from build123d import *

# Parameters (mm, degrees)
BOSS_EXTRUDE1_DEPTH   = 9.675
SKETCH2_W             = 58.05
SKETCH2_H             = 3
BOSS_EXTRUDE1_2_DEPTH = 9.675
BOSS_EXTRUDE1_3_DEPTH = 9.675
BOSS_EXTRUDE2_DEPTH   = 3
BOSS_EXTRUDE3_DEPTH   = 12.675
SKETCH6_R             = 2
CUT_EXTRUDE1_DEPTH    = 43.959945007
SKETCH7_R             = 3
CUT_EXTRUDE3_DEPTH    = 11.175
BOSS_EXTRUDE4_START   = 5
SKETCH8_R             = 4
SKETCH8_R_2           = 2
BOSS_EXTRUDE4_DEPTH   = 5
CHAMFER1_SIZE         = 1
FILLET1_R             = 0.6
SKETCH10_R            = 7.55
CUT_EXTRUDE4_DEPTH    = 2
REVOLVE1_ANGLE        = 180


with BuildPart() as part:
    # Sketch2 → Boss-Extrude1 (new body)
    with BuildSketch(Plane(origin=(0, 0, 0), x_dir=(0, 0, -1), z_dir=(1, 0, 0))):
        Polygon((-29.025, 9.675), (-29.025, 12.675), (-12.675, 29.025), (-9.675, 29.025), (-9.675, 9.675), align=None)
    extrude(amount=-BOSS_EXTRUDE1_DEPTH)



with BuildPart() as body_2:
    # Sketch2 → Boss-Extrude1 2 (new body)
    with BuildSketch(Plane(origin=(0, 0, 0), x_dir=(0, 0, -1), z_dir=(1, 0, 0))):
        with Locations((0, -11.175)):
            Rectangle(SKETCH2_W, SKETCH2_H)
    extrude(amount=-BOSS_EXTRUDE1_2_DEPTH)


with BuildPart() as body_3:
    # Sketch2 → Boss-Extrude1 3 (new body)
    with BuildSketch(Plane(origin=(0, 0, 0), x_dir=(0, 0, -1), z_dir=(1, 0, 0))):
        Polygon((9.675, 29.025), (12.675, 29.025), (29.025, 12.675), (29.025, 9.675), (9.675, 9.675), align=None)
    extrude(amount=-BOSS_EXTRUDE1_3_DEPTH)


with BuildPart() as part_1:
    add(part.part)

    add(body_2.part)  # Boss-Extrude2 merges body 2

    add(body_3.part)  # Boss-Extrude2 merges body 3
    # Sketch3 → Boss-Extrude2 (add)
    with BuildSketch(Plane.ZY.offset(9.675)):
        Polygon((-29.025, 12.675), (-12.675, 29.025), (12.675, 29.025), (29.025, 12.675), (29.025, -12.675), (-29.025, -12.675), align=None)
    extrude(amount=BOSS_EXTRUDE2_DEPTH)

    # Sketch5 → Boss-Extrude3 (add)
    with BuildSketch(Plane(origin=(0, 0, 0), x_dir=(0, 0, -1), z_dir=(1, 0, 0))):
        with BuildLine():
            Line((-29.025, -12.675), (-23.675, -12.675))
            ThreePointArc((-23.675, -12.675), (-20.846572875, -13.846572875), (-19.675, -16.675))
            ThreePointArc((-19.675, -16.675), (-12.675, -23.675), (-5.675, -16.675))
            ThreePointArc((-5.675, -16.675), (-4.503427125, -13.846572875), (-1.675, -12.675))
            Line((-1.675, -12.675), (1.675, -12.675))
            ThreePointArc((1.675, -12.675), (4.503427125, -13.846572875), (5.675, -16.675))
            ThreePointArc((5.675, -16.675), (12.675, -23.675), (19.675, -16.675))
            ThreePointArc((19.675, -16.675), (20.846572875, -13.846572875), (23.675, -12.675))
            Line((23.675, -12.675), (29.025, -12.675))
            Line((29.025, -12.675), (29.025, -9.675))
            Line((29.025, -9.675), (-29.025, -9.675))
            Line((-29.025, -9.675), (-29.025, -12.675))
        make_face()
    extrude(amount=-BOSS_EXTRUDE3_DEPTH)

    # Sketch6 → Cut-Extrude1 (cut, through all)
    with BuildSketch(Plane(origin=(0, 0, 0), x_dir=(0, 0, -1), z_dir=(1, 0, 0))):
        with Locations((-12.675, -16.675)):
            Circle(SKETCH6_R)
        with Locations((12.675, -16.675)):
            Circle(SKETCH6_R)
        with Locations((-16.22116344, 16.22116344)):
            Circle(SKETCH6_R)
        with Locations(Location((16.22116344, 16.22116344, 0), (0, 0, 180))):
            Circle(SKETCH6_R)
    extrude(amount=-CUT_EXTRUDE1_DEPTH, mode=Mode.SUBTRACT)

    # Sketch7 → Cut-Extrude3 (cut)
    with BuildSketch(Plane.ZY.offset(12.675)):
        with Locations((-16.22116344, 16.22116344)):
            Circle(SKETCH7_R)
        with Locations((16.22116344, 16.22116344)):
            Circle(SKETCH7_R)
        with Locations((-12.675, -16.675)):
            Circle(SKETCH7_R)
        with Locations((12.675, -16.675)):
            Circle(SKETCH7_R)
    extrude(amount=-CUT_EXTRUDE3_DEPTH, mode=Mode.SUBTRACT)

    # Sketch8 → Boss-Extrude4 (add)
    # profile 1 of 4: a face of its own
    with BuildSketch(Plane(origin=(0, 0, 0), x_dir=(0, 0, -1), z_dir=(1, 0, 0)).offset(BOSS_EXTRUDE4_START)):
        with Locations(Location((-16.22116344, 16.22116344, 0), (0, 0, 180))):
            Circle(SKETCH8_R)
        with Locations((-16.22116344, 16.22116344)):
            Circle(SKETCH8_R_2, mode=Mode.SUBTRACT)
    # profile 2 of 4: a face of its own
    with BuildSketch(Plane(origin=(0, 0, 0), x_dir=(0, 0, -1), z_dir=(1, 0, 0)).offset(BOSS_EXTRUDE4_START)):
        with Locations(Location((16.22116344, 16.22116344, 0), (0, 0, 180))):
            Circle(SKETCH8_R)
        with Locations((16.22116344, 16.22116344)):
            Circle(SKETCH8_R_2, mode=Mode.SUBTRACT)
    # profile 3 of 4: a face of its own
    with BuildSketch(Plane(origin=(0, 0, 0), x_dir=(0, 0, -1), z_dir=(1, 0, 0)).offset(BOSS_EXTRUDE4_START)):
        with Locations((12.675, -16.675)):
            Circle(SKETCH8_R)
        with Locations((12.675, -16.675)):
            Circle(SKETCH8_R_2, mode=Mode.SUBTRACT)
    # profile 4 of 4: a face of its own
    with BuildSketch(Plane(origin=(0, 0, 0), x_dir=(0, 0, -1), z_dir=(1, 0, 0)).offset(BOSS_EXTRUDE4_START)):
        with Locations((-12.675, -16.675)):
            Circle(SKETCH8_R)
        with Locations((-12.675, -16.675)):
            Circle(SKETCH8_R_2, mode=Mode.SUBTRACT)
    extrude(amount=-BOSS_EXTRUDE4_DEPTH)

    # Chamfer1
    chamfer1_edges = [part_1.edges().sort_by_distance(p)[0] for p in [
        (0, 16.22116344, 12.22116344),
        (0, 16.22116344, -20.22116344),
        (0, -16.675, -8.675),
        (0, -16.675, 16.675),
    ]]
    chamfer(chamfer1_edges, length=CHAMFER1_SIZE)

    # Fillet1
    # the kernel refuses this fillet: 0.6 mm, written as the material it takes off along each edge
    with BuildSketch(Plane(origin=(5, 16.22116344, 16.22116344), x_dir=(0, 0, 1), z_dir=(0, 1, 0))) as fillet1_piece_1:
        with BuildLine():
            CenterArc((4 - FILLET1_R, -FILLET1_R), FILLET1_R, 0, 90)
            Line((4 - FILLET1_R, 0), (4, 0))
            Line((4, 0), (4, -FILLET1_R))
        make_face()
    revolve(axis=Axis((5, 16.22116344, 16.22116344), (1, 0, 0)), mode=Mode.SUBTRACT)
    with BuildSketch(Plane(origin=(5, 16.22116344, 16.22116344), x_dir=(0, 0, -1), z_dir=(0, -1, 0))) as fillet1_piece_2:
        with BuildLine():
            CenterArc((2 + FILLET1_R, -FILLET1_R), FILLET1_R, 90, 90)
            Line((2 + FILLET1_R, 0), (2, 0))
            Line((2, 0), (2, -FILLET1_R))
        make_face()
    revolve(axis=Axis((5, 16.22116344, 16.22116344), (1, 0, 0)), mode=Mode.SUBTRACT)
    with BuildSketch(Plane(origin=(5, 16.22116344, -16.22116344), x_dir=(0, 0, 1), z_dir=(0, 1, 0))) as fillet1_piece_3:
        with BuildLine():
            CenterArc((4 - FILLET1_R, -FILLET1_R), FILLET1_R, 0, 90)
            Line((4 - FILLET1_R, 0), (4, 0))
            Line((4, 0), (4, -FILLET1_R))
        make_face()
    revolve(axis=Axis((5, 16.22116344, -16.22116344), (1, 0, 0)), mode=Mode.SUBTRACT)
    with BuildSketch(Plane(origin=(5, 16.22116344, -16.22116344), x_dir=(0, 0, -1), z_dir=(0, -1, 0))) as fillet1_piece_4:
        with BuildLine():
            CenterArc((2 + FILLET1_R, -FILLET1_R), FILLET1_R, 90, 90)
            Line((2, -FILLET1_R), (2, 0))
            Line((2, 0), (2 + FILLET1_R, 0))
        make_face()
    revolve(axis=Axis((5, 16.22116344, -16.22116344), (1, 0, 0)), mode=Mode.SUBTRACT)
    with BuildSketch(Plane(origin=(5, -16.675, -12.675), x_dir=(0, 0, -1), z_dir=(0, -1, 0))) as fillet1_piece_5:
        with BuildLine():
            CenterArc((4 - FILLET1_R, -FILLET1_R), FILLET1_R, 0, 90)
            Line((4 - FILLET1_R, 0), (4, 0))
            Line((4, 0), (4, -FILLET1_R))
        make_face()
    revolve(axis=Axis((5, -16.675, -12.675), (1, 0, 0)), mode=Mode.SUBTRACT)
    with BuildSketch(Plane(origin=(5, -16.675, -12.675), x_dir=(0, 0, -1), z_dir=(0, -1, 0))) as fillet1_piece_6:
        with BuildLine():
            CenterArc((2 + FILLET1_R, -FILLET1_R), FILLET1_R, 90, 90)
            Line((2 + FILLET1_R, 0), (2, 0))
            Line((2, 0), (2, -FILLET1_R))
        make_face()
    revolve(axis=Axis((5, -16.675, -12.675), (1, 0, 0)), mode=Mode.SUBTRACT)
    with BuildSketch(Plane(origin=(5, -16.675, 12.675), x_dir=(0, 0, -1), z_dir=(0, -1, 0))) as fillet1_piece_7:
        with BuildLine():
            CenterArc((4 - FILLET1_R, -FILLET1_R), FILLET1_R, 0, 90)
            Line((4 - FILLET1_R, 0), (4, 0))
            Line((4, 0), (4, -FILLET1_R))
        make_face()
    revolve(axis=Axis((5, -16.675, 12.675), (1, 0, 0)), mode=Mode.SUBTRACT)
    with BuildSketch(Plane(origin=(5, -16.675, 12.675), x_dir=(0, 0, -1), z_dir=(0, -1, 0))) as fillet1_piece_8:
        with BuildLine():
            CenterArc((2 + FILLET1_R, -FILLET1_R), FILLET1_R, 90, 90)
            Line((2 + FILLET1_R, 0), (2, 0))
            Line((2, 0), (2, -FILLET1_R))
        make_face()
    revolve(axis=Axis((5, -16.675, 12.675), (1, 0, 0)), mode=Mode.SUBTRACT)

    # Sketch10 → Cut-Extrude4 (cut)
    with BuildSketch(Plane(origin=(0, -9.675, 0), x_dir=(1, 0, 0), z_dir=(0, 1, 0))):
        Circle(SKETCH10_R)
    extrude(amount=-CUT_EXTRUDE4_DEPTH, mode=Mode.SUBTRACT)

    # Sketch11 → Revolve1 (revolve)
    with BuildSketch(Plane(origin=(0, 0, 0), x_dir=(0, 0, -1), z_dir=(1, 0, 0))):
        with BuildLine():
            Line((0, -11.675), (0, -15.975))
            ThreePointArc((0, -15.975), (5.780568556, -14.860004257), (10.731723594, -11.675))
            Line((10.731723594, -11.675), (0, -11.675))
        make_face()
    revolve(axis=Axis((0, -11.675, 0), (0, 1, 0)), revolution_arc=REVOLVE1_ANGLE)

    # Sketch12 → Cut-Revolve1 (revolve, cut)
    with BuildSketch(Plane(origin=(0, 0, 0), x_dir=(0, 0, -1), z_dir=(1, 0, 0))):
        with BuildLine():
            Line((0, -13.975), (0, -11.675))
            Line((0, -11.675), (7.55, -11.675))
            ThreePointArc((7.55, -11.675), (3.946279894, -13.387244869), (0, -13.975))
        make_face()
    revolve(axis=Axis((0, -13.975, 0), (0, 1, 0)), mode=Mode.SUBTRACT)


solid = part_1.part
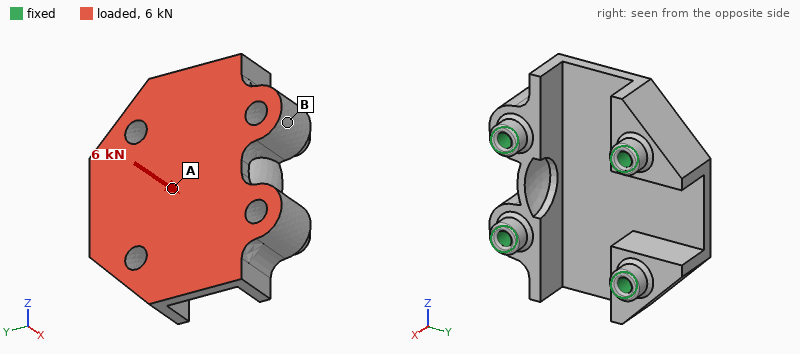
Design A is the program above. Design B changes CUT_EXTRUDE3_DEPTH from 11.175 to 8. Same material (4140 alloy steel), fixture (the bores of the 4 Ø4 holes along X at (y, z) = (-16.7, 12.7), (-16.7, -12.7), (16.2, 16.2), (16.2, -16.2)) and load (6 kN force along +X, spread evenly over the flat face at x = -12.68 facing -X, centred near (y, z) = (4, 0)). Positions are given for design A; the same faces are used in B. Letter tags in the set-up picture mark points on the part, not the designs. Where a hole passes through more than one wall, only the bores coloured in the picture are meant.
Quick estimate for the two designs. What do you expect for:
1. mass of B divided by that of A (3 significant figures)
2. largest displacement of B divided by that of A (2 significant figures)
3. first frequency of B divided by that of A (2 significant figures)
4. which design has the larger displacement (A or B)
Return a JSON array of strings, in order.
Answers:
["1.01", "0.92", "1.5", "A"]
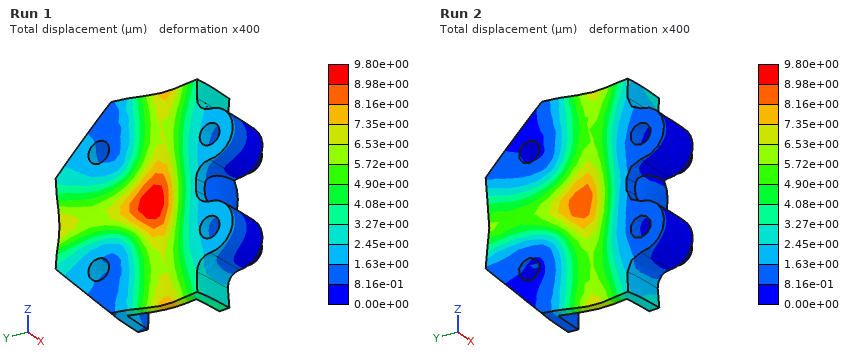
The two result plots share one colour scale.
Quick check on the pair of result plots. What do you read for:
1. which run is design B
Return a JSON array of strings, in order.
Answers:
["Run 2"]
